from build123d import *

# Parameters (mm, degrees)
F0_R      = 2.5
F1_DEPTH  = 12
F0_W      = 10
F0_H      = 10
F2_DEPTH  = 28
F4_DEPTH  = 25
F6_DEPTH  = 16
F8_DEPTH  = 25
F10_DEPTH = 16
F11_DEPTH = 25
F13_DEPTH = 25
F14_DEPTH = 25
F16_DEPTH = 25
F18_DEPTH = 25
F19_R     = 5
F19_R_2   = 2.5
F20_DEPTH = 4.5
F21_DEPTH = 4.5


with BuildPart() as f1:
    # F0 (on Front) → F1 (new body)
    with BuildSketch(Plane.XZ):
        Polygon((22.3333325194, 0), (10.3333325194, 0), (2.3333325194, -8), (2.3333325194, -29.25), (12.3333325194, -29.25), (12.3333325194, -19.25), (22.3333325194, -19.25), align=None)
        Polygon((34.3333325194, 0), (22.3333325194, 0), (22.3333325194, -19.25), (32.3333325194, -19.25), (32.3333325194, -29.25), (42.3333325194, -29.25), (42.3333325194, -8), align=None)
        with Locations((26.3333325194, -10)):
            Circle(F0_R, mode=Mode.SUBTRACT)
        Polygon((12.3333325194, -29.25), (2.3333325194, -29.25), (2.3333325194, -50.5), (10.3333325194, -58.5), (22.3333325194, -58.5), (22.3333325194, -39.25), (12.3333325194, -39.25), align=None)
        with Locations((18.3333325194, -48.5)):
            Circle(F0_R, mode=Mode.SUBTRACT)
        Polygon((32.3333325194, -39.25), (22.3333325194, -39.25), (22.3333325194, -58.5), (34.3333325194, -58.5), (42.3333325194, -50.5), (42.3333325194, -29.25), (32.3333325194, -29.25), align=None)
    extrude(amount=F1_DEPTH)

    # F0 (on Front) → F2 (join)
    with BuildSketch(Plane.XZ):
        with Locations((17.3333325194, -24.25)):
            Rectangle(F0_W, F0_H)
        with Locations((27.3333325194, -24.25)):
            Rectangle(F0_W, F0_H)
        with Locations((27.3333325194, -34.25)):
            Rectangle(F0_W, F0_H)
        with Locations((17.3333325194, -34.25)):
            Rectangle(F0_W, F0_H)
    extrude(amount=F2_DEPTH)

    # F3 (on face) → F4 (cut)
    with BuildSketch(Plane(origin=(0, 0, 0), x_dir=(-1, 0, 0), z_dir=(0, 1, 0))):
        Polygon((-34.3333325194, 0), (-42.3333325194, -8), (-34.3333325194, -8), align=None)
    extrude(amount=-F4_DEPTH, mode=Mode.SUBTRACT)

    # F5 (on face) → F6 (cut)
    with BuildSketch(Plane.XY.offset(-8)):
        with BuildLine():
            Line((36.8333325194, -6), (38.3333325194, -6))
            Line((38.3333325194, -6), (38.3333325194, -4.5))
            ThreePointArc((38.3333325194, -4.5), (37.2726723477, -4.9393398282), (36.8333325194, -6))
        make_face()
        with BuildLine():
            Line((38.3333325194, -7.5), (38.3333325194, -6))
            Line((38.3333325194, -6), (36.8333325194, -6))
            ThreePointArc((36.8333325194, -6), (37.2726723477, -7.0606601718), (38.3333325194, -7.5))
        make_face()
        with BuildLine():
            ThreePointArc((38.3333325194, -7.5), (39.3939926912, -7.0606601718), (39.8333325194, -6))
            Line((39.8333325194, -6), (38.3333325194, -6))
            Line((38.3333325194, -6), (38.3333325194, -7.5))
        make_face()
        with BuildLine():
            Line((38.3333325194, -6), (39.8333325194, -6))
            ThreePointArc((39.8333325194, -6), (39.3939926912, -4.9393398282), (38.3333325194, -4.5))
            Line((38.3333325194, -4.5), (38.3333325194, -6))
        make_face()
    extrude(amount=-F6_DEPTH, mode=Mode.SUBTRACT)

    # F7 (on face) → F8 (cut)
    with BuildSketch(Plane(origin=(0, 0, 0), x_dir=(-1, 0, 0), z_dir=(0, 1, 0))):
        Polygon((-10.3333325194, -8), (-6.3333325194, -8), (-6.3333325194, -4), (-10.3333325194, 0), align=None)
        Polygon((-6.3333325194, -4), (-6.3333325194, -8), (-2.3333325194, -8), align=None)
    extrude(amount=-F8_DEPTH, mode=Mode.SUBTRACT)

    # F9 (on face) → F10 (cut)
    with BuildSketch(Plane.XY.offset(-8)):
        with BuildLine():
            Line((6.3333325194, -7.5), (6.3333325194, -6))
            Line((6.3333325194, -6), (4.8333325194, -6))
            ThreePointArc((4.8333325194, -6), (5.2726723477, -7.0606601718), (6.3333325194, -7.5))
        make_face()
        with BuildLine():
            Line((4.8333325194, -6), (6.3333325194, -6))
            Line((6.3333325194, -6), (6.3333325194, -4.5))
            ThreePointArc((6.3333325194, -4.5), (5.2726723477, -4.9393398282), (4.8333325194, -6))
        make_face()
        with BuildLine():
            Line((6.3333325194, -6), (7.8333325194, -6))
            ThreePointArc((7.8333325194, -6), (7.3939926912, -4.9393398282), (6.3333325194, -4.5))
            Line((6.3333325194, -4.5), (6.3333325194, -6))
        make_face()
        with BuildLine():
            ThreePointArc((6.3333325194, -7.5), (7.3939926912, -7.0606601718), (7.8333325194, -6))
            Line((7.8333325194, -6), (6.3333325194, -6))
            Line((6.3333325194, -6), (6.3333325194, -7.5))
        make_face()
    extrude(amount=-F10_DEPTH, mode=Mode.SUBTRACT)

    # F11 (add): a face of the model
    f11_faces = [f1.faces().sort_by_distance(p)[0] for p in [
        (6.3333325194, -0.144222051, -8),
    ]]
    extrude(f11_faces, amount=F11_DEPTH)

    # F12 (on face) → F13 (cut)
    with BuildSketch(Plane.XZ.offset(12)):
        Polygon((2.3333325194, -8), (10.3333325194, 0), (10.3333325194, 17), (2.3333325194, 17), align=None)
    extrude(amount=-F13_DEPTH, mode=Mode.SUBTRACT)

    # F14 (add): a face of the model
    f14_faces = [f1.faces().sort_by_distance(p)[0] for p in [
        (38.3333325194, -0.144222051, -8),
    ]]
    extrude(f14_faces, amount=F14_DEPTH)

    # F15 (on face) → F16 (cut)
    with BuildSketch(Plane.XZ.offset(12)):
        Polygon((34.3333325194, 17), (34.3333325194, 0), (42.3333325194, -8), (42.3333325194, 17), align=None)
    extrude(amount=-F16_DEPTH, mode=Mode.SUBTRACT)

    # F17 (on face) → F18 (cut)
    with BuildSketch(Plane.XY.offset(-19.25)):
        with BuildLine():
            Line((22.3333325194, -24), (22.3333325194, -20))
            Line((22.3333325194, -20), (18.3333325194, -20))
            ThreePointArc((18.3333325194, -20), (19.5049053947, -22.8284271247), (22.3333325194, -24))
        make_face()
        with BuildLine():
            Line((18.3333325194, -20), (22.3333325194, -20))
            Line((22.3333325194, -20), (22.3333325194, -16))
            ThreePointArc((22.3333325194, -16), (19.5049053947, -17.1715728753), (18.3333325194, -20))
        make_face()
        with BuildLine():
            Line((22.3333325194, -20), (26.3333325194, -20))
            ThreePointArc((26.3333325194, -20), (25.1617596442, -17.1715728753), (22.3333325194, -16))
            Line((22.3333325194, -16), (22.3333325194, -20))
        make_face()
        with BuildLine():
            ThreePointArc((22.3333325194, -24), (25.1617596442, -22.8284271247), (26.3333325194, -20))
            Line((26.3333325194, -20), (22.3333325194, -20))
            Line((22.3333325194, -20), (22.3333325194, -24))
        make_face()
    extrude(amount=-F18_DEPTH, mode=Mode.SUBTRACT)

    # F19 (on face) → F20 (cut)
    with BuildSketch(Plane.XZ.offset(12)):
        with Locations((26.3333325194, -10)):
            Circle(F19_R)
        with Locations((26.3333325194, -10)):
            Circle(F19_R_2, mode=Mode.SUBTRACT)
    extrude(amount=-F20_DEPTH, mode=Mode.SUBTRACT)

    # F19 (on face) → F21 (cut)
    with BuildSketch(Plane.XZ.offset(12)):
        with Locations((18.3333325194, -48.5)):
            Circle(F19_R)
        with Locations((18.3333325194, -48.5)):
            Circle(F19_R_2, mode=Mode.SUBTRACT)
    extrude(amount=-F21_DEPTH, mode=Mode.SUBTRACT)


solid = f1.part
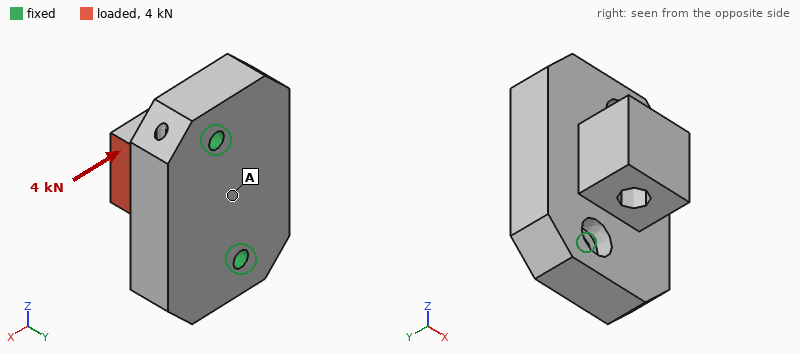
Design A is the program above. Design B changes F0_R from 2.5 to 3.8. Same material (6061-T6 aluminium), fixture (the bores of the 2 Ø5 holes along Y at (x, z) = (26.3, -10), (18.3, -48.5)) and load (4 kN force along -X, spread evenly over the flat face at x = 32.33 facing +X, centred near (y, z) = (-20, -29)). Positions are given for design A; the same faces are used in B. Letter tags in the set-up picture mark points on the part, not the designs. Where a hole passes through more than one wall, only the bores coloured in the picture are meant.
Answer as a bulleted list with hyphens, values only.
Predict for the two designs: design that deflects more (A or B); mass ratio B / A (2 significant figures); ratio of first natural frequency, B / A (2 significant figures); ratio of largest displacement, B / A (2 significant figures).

- A
- 0.99
- 1.3
- 0.71
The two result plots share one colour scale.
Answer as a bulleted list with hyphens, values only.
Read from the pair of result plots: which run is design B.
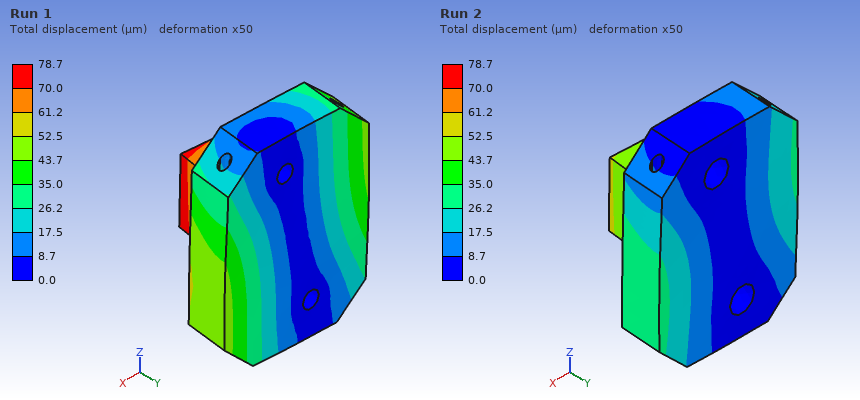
- Run 2
